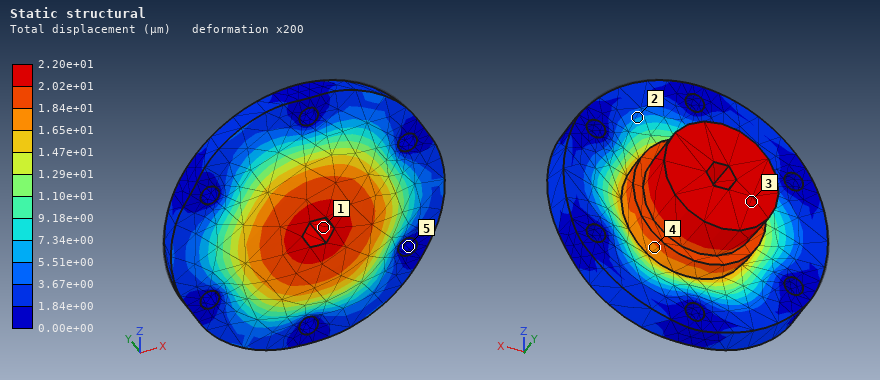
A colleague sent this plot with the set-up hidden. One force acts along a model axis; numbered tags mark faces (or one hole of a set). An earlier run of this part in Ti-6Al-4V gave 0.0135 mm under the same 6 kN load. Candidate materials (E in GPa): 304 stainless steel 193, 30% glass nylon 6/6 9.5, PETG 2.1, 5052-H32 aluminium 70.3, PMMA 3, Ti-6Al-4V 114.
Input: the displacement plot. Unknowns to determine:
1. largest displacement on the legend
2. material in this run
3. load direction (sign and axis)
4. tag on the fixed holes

2.20e+01 µm
5052-H32 aluminium
-Y
5
